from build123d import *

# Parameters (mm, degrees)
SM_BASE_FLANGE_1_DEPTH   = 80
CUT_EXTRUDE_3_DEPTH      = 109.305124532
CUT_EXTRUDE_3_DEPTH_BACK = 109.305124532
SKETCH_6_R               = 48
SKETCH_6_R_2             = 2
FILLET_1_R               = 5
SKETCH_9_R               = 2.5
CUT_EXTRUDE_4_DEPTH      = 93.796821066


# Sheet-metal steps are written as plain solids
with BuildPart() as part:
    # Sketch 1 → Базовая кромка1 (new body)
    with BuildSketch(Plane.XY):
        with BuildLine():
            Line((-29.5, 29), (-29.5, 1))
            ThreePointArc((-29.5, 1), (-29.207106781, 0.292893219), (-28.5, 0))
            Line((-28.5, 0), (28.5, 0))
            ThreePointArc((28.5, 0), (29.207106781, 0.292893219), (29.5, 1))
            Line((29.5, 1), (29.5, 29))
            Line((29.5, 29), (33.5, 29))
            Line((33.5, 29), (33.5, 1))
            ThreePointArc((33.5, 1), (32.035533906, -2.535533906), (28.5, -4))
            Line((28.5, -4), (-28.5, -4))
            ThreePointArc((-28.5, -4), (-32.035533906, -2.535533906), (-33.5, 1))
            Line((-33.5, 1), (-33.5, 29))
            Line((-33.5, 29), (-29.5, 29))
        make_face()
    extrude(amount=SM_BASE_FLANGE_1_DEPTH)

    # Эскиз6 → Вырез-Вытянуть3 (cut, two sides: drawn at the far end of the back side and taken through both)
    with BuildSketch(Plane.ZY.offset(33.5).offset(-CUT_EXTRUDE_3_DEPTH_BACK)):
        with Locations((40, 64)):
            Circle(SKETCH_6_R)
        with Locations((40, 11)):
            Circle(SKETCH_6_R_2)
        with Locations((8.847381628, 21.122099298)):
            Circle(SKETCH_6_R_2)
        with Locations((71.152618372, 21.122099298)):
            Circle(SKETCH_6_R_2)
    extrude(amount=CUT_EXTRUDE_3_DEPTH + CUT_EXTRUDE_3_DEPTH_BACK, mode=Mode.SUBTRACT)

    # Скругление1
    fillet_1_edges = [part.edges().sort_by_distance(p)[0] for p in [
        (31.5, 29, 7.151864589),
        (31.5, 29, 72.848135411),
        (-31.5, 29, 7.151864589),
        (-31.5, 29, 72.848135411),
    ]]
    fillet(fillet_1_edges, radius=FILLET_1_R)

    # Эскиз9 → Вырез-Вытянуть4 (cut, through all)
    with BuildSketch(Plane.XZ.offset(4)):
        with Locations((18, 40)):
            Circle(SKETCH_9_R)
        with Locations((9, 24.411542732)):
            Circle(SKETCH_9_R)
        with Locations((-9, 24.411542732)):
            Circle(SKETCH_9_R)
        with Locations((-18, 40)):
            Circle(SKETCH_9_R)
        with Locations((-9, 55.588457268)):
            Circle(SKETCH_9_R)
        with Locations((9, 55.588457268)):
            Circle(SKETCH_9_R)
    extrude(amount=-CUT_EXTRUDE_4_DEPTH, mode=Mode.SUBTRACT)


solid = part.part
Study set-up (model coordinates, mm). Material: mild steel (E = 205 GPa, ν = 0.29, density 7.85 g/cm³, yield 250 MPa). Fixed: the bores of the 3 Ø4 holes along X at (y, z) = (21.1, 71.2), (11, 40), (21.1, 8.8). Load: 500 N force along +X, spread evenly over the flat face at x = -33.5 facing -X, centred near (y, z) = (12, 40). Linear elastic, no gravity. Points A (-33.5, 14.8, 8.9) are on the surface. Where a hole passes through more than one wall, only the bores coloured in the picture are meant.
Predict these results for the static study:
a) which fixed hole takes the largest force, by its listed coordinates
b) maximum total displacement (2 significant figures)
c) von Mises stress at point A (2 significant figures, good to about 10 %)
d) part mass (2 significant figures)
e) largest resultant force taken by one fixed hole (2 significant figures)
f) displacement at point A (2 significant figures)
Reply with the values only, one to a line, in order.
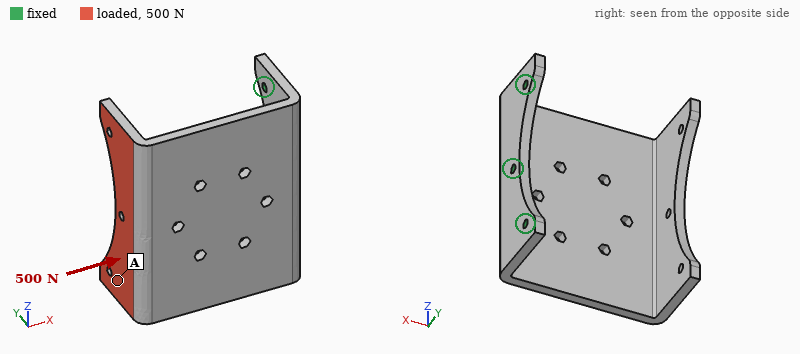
(11, 40)
0.26 mm
6.6 MPa
260 g
280 N
0.21 mm
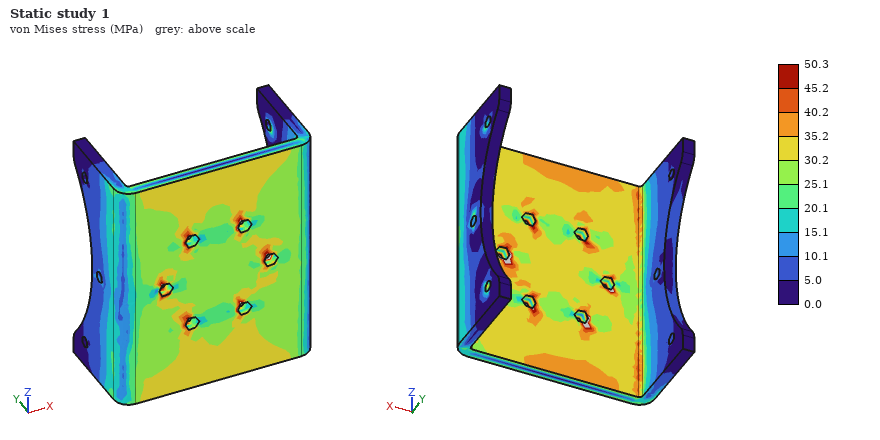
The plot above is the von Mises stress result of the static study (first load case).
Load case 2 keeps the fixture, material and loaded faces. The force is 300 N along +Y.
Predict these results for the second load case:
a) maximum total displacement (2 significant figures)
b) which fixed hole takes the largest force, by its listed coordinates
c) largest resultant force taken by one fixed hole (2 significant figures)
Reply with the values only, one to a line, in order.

0.61 mm
(11, 40)
540 N
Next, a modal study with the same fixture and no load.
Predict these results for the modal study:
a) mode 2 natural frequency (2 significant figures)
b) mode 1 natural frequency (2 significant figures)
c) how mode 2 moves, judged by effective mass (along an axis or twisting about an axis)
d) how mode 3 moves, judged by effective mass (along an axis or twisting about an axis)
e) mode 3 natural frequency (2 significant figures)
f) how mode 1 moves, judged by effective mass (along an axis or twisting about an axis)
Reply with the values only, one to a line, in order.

790 Hz
390 Hz
along Z
along Z
1400 Hz
along Y
